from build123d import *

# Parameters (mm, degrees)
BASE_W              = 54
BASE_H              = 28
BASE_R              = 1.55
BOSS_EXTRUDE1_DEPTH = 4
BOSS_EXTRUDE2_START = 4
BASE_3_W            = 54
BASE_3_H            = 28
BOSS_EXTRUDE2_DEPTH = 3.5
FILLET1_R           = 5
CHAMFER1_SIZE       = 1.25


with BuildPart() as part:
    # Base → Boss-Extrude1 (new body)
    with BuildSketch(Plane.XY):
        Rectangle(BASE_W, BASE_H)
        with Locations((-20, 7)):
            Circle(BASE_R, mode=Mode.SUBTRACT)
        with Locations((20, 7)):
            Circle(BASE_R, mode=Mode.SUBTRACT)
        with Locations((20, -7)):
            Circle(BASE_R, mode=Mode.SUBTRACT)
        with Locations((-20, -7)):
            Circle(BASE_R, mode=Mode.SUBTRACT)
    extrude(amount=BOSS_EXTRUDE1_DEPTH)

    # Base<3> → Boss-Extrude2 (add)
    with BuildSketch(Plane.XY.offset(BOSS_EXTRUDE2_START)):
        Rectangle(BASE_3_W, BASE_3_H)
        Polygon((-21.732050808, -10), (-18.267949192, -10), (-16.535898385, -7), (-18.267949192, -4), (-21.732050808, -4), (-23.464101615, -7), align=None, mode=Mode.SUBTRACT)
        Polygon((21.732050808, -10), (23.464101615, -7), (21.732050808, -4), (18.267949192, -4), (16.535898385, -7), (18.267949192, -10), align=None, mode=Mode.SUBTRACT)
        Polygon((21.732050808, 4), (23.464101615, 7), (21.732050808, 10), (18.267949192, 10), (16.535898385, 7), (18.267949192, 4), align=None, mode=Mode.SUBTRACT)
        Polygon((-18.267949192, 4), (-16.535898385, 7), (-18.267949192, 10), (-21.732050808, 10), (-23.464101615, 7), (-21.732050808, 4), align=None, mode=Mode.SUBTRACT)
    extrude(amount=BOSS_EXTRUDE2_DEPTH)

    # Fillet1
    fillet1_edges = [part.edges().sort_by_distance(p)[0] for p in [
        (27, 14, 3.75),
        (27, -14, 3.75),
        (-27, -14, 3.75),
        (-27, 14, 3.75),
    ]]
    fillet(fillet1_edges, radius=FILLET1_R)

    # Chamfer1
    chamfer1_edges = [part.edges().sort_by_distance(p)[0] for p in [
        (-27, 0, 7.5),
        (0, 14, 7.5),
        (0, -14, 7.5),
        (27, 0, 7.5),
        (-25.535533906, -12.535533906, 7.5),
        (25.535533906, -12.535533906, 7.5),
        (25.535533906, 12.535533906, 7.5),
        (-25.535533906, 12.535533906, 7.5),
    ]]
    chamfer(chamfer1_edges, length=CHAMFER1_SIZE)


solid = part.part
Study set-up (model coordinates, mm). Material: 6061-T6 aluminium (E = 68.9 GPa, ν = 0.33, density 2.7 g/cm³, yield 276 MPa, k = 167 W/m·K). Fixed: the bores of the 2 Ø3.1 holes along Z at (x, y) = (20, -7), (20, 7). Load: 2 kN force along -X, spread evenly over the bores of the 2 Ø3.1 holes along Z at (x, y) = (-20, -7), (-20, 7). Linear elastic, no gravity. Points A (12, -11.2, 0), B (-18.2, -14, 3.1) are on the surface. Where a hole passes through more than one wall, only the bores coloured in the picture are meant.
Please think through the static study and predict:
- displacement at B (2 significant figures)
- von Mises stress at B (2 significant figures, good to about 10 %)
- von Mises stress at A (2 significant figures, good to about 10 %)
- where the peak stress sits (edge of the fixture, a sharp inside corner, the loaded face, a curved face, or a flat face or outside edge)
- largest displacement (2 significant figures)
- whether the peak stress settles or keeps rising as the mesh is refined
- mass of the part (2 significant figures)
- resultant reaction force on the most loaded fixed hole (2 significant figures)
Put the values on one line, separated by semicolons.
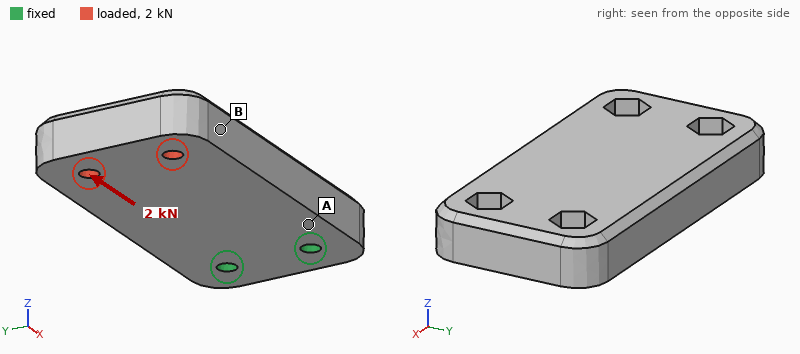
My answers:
32 µm; 5.8 MPa; 22 MPa; edge of the fixture; 51 µm; keeps rising; 28 g; 1.0 kN
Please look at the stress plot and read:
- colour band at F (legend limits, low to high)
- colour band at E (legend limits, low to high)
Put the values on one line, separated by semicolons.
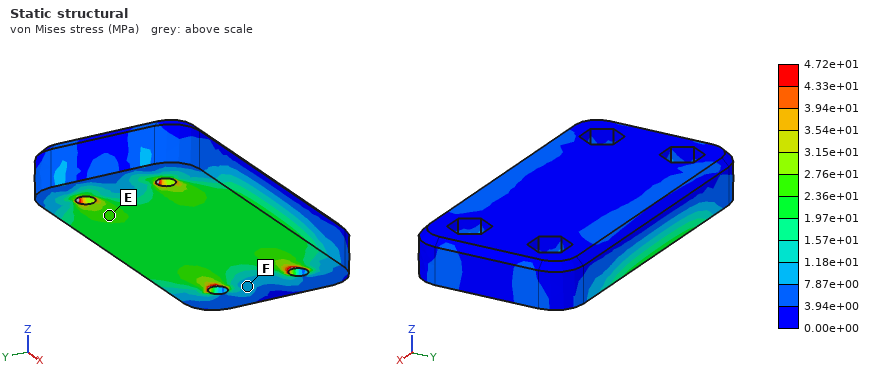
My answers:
7.87e+00 to 1.18e+01 MPa; 2.36e+01 to 2.76e+01 MPa
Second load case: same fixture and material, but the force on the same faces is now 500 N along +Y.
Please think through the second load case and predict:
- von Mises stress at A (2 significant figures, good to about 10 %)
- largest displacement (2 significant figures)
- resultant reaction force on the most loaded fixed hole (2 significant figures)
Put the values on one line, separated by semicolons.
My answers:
17 MPa; 35 µm; 1.3 kN
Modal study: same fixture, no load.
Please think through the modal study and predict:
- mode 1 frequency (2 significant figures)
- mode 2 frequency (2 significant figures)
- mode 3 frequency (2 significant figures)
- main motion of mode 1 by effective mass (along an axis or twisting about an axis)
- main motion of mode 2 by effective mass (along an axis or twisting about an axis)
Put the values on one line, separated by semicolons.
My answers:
2100 Hz; 6600 Hz; 8400 Hz; along Z; along Y
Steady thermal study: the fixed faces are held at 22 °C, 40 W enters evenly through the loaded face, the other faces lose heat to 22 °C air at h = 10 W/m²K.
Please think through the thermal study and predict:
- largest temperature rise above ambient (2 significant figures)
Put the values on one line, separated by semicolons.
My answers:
55 K
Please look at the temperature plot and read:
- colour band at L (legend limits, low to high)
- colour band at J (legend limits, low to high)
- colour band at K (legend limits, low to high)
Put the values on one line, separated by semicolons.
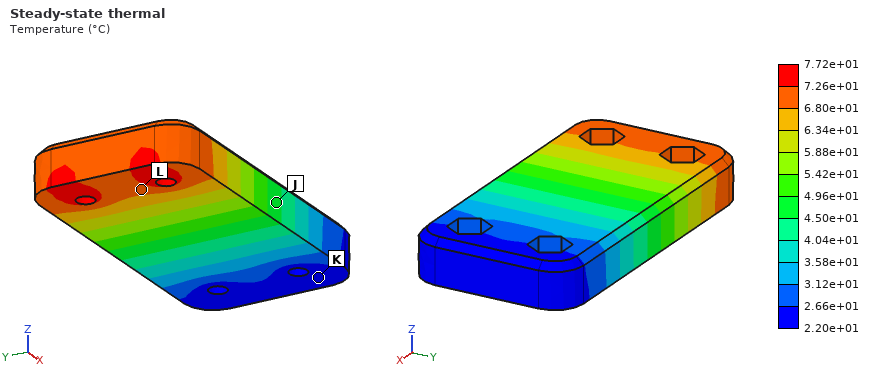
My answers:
6.80e+01 to 7.26e+01 °C; 4.50e+01 to 4.96e+01 °C; 2.20e+01 to 2.66e+01 °C
